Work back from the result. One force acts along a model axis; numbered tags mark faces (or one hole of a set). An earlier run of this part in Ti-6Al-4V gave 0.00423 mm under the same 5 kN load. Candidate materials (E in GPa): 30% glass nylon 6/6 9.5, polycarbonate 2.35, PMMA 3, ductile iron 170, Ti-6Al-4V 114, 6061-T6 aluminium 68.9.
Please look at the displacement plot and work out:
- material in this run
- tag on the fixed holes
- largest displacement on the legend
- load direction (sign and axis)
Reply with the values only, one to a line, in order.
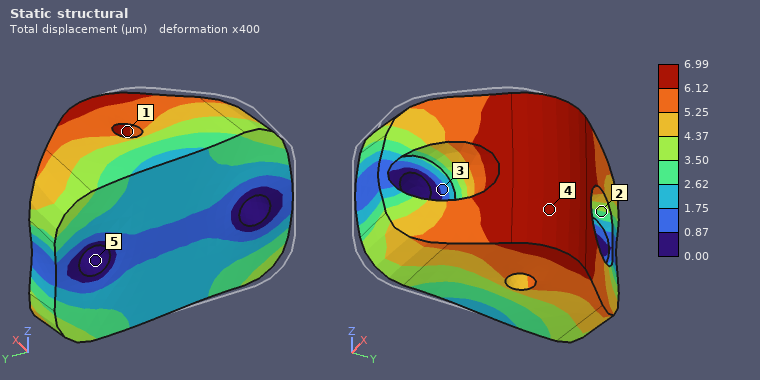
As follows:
6061-T6 aluminium
5
6.99 µm
+Y
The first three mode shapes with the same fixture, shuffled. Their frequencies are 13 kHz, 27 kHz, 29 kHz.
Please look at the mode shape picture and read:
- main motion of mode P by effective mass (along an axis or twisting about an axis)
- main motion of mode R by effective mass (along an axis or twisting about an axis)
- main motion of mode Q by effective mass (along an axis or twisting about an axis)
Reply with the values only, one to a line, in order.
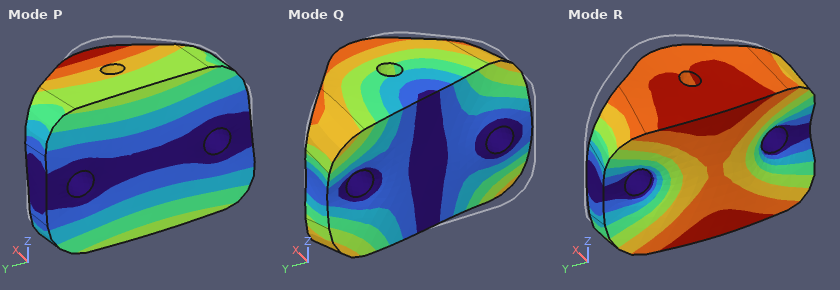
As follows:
along Z
along X
along Y
